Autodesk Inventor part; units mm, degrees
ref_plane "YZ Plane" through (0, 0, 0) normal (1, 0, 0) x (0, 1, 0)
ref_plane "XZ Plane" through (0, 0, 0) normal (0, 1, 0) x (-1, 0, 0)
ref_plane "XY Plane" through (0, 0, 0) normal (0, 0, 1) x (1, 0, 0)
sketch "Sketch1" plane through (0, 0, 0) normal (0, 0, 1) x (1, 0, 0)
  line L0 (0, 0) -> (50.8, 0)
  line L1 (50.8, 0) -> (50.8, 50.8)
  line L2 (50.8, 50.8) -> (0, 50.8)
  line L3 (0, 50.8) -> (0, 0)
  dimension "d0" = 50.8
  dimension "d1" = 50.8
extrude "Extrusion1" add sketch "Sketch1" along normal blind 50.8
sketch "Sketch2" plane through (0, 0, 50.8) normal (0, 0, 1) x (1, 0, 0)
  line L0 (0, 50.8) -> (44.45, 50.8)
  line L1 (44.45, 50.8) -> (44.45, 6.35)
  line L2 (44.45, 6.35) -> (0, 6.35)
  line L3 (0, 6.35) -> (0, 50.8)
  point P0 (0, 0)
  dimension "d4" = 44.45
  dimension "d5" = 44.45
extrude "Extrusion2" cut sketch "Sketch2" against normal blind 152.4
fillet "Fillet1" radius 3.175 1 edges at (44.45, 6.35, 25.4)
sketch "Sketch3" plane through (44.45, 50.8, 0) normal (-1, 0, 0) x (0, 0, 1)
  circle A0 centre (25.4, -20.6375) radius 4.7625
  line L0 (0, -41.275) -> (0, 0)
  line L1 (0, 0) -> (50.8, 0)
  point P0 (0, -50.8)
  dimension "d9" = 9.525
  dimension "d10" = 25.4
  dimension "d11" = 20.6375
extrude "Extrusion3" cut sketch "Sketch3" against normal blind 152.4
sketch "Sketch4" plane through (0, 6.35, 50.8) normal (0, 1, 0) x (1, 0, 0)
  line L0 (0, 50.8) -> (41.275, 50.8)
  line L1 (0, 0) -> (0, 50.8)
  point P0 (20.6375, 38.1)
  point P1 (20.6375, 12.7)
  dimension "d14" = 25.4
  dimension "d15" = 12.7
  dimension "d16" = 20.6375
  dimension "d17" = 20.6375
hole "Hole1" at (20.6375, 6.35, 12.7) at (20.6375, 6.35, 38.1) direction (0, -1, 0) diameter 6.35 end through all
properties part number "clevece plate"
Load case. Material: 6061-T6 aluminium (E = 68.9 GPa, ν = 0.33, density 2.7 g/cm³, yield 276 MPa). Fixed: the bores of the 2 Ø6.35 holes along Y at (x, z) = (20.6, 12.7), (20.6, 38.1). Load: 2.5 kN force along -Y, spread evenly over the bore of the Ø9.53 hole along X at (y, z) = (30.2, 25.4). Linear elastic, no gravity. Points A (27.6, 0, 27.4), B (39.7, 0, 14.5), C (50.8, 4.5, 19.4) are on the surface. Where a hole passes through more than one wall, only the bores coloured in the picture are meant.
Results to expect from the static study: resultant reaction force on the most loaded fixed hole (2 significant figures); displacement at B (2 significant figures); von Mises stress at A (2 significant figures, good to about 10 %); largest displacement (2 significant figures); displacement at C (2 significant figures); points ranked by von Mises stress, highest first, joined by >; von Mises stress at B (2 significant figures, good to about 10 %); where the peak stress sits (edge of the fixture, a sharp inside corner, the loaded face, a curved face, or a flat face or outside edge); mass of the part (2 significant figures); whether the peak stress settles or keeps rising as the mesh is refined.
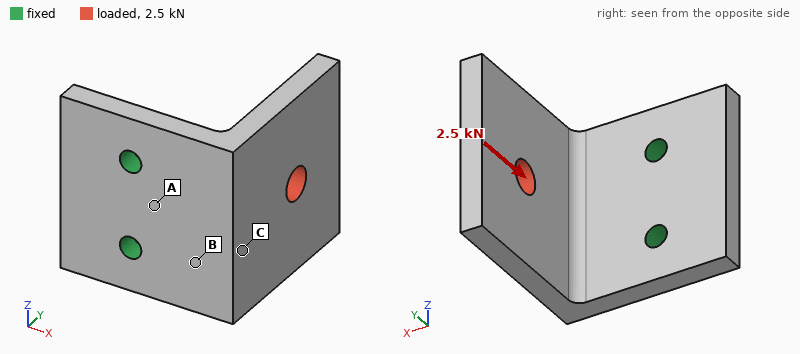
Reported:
1.3 kN
0.12 mm
110 MPa
0.58 mm
0.24 mm
A > B > C
51 MPa
edge of the fixture
81 g
keeps rising
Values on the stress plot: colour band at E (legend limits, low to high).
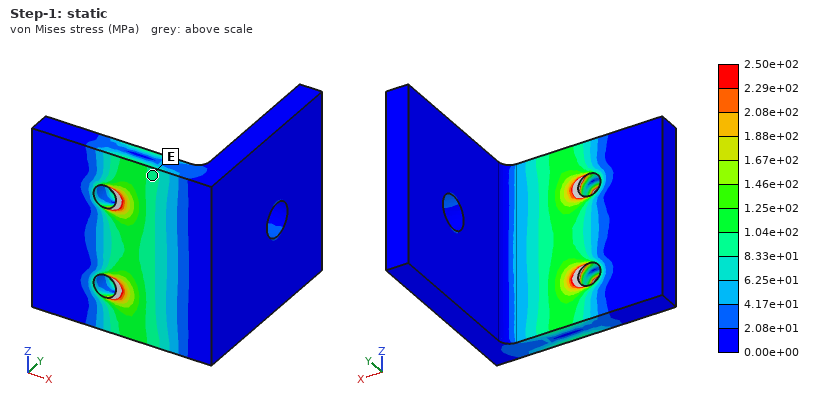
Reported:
8.33e+01 to 1.04e+02 MPa
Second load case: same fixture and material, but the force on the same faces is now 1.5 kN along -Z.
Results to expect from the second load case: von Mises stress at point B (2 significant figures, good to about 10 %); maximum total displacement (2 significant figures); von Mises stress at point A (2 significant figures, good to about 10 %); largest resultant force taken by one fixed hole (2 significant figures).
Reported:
42 MPa
0.25 mm
27 MPa
1.9 kN
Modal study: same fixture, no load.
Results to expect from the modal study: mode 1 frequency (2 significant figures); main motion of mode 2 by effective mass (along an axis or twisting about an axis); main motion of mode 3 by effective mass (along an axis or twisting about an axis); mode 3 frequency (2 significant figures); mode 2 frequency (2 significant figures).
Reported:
1300 Hz
along Z
along Y
4100 Hz
2300 Hz
